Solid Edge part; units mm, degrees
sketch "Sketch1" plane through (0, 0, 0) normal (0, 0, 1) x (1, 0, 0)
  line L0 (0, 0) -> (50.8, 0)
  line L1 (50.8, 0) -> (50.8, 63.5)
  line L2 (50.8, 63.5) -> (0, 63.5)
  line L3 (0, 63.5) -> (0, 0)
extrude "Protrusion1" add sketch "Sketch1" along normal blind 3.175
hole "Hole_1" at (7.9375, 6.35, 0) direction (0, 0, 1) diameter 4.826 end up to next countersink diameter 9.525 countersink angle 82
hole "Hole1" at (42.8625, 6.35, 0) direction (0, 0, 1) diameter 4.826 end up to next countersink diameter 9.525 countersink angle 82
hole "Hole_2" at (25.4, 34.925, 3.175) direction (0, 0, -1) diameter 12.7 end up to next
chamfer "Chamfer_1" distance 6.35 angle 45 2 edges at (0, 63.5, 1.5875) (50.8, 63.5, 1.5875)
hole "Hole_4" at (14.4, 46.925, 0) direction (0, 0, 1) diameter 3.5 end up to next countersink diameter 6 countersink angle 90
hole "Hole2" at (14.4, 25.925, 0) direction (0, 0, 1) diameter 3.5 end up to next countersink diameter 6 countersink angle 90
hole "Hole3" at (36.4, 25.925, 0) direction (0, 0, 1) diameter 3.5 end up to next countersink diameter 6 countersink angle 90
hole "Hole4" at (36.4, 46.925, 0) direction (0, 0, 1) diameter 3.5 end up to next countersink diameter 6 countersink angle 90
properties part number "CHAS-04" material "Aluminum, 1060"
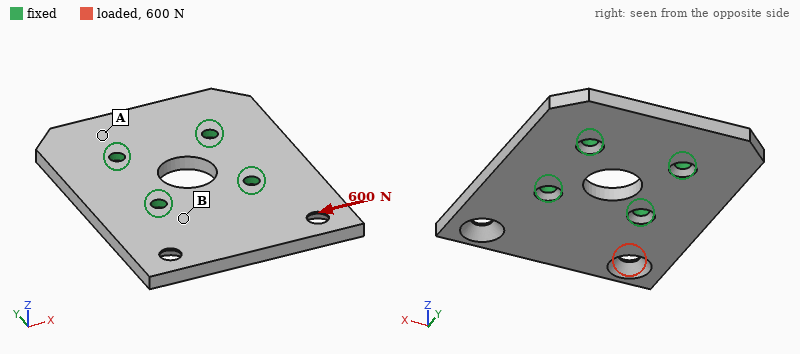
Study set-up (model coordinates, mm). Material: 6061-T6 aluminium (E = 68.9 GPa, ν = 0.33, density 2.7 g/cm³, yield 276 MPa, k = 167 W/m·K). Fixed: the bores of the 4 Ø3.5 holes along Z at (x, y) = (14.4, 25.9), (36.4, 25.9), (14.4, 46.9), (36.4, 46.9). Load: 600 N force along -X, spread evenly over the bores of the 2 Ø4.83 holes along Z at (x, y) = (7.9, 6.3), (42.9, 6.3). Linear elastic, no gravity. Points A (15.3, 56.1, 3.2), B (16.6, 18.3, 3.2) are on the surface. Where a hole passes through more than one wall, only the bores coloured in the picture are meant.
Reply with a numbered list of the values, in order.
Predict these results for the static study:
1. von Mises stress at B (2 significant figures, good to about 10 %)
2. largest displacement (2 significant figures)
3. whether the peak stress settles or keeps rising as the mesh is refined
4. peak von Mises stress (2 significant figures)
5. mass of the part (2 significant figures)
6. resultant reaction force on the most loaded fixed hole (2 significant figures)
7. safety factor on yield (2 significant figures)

1. 14 MPa
2. 26 µm
3. settles
4. 89 MPa
5. 25 g
6. 440 N
7. 3.1
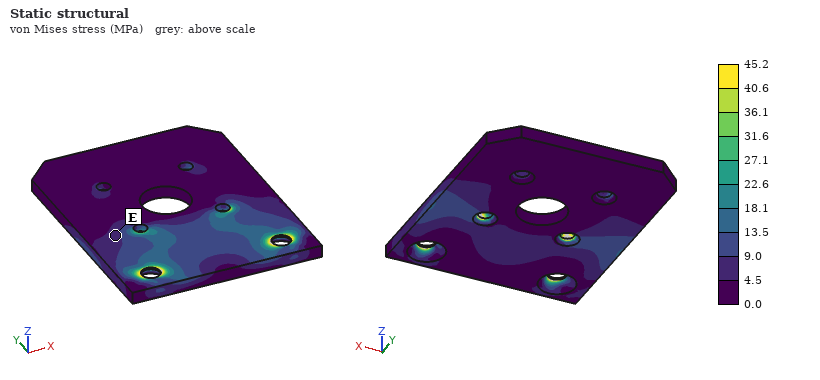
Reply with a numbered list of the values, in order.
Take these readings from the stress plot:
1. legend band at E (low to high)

1. 4.5 to 9.0 MPa
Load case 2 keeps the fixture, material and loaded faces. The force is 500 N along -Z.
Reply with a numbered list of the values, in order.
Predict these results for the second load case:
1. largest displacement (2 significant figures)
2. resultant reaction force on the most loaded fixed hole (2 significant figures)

1. 0.29 mm
2. 420 N
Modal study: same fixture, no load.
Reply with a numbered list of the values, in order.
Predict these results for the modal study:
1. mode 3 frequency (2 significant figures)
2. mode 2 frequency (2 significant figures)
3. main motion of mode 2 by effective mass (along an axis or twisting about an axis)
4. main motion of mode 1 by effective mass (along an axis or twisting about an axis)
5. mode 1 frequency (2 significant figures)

1. 7700 Hz
2. 5000 Hz
3. twisting about Y
4. along Z
5. 3400 Hz
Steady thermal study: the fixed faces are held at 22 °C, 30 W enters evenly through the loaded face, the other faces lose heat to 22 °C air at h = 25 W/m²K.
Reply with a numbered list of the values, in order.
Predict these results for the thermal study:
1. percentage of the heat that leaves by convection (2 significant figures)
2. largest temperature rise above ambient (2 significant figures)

1. 5.1 %
2. 43 K
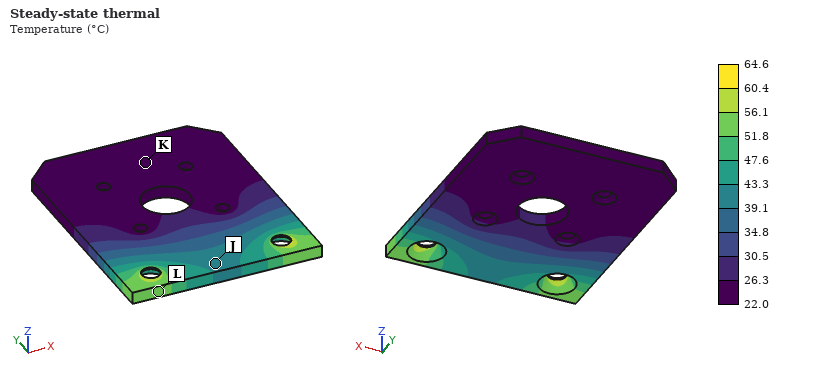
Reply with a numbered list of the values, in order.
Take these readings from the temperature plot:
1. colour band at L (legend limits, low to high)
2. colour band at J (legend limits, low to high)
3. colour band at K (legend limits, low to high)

1. 51.8 to 56.1 °C
2. 39.1 to 43.3 °C
3. 22.0 to 26.3 °C
